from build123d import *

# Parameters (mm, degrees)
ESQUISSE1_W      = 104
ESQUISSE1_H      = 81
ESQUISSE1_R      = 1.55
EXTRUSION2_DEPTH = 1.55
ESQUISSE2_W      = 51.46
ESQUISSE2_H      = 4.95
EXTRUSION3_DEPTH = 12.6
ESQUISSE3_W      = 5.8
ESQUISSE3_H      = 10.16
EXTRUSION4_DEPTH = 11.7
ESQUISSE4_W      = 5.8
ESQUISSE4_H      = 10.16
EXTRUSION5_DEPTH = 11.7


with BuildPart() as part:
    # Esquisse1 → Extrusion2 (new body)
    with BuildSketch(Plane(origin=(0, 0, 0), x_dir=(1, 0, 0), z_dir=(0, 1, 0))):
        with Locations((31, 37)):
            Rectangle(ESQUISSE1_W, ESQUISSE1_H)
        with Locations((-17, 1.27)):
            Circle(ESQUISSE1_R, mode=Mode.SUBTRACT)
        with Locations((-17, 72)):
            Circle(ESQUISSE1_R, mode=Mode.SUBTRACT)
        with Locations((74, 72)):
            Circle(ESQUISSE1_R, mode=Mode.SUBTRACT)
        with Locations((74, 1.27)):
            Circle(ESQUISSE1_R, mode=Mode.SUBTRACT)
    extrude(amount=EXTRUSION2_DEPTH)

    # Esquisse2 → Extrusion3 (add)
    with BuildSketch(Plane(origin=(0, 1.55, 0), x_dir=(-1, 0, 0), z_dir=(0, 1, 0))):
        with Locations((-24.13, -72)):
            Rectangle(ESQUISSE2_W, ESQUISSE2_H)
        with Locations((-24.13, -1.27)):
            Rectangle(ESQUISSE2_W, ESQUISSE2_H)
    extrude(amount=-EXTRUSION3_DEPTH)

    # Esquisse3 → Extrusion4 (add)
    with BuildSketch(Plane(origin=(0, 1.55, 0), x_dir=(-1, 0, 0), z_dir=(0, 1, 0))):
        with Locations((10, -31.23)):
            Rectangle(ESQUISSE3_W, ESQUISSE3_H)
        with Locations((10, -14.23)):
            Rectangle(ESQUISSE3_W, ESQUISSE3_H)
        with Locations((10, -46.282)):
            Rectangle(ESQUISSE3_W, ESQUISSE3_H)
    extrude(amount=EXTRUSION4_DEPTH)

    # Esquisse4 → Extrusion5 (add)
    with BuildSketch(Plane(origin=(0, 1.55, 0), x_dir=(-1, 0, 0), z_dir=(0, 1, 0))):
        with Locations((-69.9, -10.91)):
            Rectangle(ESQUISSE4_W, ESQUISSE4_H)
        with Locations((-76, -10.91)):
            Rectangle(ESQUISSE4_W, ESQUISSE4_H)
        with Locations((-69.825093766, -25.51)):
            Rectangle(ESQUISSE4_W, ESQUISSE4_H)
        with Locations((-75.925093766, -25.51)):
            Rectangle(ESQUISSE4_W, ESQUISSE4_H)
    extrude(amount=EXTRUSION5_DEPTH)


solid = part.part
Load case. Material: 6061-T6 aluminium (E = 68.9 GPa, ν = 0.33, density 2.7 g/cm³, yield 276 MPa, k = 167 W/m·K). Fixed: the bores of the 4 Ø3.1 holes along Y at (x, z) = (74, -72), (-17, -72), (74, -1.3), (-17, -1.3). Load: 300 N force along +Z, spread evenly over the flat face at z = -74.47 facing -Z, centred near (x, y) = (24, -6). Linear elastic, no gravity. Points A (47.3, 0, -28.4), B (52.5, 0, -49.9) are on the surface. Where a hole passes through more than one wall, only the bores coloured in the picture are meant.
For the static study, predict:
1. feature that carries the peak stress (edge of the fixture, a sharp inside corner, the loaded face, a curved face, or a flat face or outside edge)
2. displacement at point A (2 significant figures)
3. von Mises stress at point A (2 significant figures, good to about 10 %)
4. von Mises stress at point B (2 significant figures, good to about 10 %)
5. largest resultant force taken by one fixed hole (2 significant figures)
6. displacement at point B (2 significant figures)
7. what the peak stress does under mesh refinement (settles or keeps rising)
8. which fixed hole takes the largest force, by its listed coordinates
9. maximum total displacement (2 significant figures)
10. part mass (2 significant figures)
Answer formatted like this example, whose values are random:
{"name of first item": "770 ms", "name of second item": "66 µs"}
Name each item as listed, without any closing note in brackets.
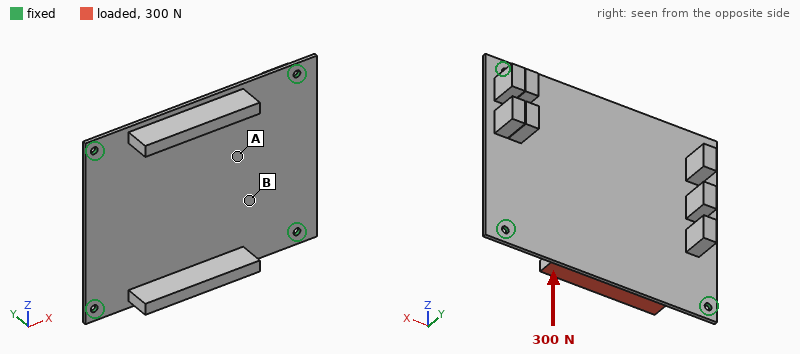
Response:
{"feature that carries the peak stress": "edge of the fixture", "displacement at point A": "0.084 mm", "von Mises stress at point A": "6.1 MPa", "von Mises stress at point B": "17 MPa", "largest resultant force taken by one fixed hole": "100 N", "displacement at point B": "0.083 mm", "what the peak stress does under mesh refinement": "keeps rising", "which fixed hole takes the largest force, by its listed coordinates": "(-17, -72)", "maximum total displacement": "0.19 mm", "part mass": "63 g"}
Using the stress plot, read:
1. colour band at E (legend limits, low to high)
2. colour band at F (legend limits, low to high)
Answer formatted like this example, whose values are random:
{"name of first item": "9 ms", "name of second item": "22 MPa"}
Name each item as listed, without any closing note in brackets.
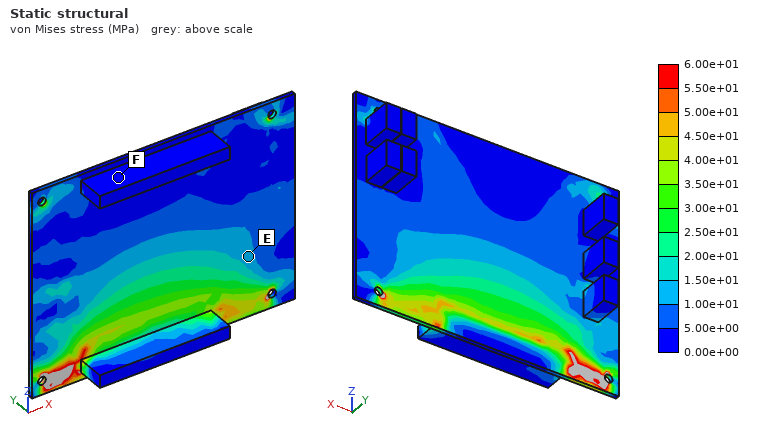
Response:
{"colour band at E": "1.00e+01 to 1.50e+01 MPa", "colour band at F": "0.00e+00 to 5.00e+00 MPa"}
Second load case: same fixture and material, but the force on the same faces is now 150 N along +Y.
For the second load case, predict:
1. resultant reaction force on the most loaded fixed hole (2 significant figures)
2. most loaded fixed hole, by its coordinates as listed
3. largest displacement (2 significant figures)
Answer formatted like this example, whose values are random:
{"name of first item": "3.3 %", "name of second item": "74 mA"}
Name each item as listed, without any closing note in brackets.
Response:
{"resultant reaction force on the most loaded fixed hole": "110 N", "most loaded fixed hole, by its coordinates as listed": "(-17, -72)", "largest displacement": "0.25 mm"}
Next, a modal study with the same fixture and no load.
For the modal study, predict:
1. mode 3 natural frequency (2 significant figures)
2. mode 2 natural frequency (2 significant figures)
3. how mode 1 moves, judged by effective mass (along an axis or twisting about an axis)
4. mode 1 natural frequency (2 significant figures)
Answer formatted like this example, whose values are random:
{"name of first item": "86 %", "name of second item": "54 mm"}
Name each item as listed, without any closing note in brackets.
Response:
{"mode 3 natural frequency": "1400 Hz", "mode 2 natural frequency": "1300 Hz", "how mode 1 moves, judged by effective mass": "along Y", "mode 1 natural frequency": "910 Hz"}
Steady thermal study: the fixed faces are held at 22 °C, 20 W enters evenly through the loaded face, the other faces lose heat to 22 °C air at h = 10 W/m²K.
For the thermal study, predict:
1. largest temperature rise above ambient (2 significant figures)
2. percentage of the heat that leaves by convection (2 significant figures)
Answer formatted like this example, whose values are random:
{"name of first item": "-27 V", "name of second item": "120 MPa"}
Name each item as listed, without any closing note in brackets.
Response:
{"largest temperature rise above ambient": "37 K", "percentage of the heat that leaves by convection": "14 %"}
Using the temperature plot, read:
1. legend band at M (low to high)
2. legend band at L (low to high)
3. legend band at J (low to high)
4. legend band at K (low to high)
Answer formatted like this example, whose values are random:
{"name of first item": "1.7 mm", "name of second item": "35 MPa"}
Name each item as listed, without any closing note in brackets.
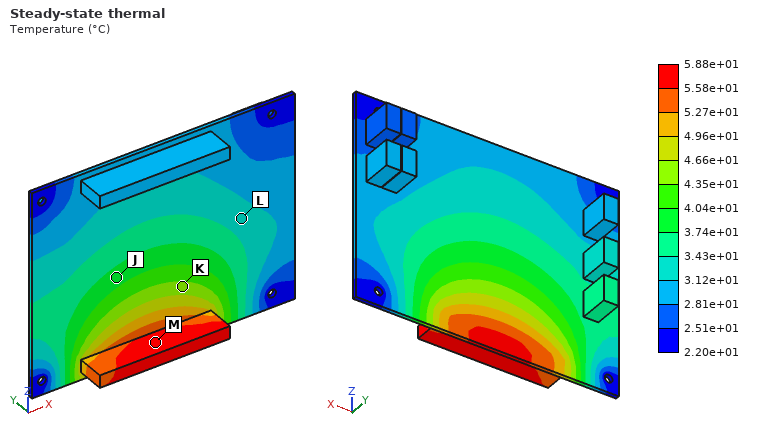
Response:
{"legend band at M": "5.58e+01 to 5.88e+01 °C", "legend band at L": "3.12e+01 to 3.43e+01 °C", "legend band at J": "3.74e+01 to 4.04e+01 °C", "legend band at K": "4.35e+01 to 4.66e+01 °C"}
